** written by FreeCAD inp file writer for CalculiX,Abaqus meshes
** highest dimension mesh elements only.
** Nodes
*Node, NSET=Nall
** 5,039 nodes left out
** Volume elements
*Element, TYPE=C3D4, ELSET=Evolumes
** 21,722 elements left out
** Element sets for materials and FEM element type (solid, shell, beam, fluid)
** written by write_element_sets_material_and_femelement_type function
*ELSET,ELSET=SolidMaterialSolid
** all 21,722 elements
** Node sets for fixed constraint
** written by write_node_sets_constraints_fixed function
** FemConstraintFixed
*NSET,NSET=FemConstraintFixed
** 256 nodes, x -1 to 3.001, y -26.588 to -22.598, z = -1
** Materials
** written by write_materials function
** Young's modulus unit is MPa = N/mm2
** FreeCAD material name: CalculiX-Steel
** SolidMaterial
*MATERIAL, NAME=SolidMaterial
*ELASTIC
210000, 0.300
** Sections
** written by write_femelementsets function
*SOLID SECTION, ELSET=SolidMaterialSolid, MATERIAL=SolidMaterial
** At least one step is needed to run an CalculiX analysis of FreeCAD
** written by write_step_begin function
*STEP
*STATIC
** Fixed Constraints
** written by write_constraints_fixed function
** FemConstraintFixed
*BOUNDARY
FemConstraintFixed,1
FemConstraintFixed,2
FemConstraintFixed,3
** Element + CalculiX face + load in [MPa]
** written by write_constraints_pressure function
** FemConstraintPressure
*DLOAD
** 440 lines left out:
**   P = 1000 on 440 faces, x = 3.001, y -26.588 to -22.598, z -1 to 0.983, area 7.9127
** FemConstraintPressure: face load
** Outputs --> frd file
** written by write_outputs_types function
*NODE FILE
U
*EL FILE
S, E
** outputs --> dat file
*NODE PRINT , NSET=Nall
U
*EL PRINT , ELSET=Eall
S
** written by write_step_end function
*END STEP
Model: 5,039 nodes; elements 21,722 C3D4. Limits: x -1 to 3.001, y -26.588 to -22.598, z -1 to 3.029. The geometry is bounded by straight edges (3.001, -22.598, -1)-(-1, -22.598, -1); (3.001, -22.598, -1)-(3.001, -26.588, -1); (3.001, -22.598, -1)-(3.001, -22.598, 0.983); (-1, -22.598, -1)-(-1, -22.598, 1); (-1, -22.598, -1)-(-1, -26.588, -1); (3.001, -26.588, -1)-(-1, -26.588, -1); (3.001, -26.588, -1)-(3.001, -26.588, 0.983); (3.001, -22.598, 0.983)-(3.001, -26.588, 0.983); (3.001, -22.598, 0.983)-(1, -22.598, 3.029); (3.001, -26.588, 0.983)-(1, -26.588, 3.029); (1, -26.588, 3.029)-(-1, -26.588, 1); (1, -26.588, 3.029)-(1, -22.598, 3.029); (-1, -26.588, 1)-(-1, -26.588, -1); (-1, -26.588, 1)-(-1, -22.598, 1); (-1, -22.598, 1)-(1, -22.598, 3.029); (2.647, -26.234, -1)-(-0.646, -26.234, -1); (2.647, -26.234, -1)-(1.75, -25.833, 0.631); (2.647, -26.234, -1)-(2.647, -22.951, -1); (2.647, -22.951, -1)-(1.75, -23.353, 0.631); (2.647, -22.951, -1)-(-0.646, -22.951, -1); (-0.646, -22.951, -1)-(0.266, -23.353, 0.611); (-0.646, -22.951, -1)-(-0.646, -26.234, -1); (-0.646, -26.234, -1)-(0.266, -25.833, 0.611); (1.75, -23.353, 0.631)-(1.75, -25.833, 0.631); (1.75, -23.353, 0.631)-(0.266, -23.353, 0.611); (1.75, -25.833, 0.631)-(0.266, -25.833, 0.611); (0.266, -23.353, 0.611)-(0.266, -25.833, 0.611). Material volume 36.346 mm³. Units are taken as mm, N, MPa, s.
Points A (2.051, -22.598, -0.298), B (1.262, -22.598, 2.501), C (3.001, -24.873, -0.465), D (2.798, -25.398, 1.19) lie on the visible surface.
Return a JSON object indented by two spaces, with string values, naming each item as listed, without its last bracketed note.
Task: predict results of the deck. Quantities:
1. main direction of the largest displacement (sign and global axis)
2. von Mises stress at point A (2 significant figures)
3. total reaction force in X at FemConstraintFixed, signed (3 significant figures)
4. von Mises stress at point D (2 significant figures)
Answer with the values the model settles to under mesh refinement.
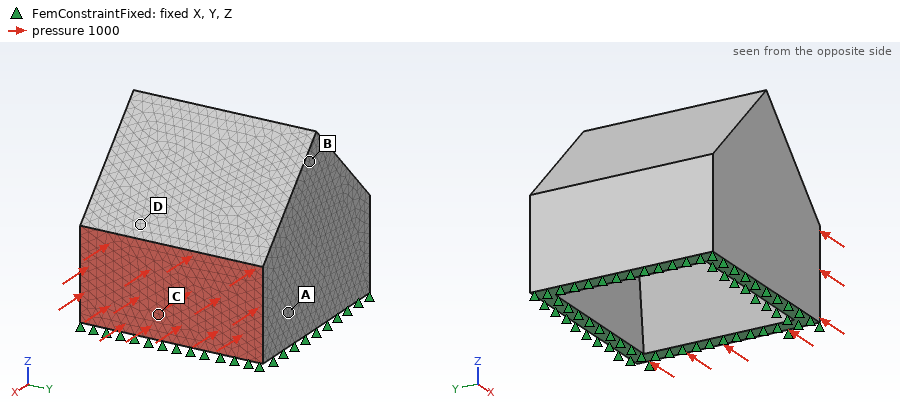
{
  "main direction of the largest displacement": "-X",
  "von Mises stress at point A": "2000 MPa",
  "total reaction force in X at FemConstraintFixed, signed": "7910 N",
  "von Mises stress at point D": "590 MPa"
}
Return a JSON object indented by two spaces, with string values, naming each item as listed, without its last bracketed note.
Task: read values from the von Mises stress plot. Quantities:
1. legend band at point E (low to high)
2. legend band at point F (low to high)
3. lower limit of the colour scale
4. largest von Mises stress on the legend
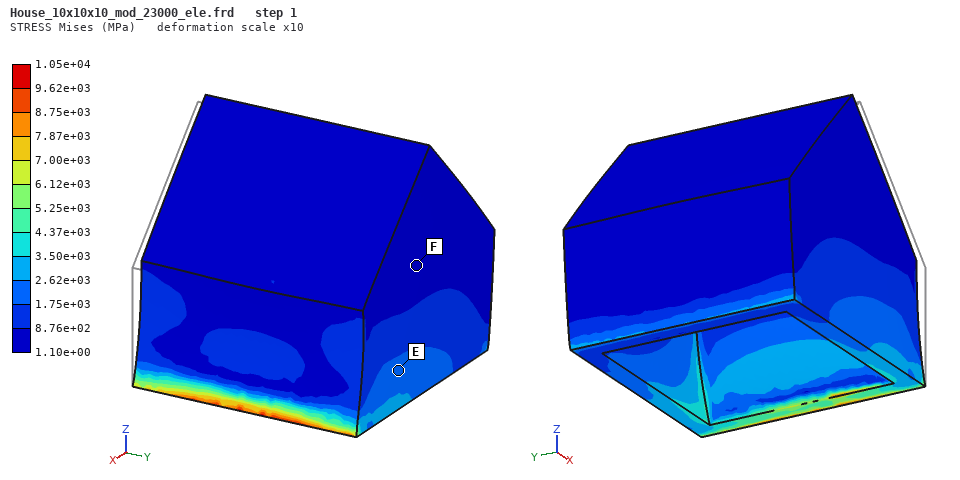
{
  "legend band at point E": "1.75e+03 to 2.62e+03 MPa",
  "legend band at point F": "1.10e+00 to 8.76e+02 MPa",
  "lower limit of the colour scale": "1.10e+00 MPa",
  "largest von Mises stress on the legend": "1.05e+04 MPa"
}
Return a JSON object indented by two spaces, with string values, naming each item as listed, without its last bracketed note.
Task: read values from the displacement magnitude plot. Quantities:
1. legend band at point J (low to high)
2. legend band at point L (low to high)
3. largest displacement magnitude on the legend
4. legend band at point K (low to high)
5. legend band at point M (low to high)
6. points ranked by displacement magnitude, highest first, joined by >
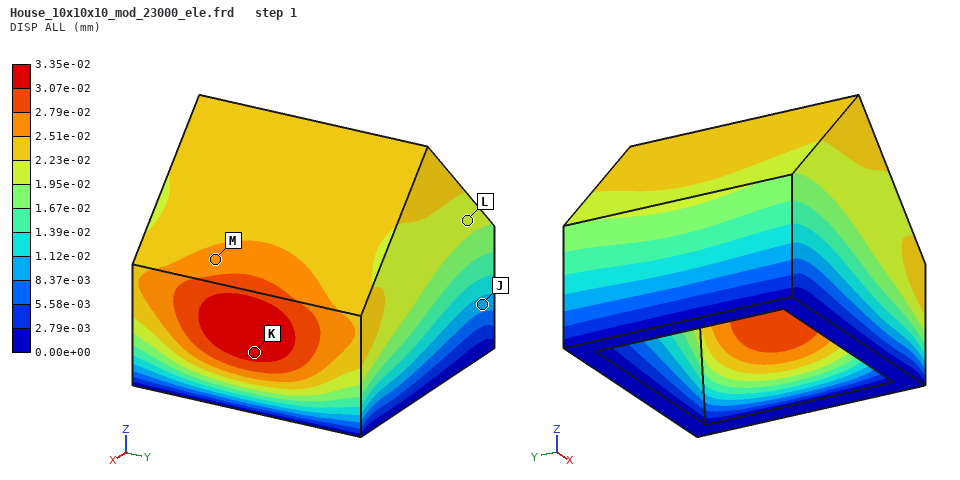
{
  "legend band at point J": "8.37e-03 to 1.12e-02 mm",
  "legend band at point L": "1.95e-02 to 2.23e-02 mm",
  "largest displacement magnitude on the legend": "3.35e-02 mm",
  "legend band at point K": "3.07e-02 to 3.35e-02 mm",
  "legend band at point M": "2.51e-02 to 2.79e-02 mm",
  "points ranked by displacement magnitude, highest first, joined by >": "K > M > L > J"
}
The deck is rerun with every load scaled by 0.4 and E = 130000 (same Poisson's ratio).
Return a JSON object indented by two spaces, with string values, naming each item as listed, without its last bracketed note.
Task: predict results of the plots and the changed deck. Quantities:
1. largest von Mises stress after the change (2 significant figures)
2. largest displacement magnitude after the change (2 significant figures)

{
  "largest von Mises stress after the change": "4200 MPa",
  "largest displacement magnitude after the change": "0.022 mm"
}
